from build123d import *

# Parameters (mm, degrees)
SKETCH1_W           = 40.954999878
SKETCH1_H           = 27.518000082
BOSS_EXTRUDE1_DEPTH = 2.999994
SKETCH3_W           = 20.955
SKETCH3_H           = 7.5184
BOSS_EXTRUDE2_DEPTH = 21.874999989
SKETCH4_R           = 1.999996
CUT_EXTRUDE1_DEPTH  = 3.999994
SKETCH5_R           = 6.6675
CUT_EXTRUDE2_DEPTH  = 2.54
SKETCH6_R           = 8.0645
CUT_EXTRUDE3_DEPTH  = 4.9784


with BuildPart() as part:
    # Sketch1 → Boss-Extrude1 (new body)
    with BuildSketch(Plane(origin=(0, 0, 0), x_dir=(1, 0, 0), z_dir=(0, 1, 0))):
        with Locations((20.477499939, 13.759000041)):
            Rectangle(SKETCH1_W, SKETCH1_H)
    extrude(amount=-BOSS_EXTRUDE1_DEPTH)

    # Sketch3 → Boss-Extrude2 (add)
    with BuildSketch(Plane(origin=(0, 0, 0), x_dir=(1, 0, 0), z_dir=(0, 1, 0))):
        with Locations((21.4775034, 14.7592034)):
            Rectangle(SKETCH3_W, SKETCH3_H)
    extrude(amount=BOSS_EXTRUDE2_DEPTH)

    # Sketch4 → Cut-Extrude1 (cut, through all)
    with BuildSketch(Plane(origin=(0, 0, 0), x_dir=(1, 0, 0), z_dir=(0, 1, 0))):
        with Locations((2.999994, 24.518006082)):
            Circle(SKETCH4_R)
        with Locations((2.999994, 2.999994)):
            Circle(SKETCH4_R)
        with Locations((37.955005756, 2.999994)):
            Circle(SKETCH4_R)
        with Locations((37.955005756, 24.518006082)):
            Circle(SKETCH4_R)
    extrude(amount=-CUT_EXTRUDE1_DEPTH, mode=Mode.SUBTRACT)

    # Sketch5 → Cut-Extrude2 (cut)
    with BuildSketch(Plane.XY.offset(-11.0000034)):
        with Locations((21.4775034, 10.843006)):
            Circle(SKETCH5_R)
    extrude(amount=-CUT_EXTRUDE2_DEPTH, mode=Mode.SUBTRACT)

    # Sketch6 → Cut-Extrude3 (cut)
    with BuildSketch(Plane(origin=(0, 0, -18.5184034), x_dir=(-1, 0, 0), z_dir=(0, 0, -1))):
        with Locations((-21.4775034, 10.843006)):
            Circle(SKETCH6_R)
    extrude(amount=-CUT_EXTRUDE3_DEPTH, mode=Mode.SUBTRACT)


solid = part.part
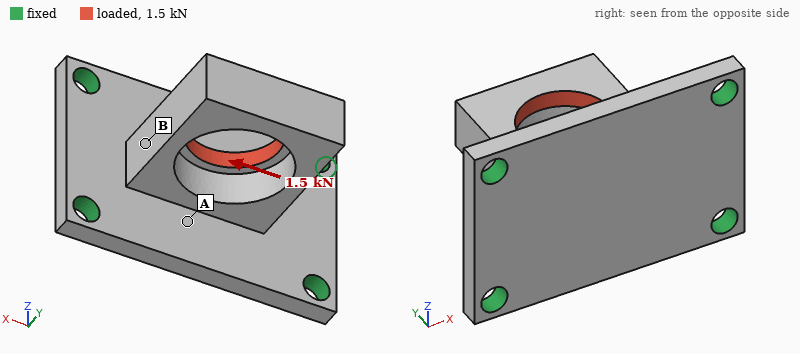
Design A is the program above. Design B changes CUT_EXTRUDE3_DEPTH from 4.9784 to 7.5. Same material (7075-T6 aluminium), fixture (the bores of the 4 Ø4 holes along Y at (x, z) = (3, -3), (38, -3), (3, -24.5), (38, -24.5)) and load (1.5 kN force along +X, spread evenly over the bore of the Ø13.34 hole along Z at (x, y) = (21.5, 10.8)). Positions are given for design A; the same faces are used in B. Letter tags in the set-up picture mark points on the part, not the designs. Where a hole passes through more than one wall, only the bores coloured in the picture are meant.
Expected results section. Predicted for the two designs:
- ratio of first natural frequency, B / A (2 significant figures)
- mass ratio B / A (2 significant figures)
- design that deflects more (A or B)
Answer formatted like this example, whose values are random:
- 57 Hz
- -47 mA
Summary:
- 1.0
- 0.97
- B
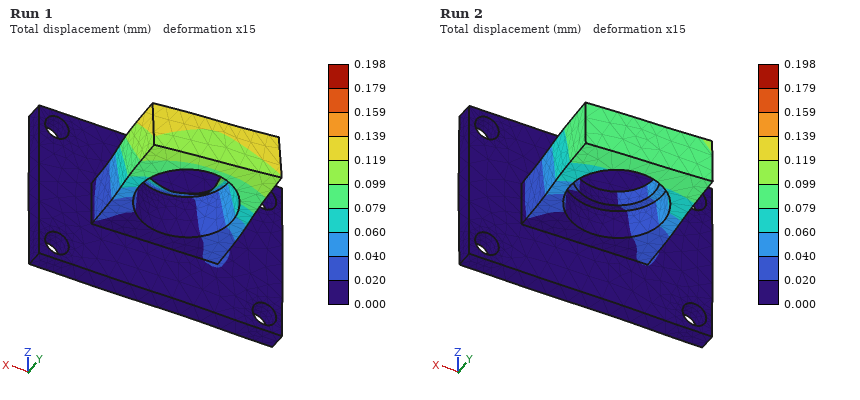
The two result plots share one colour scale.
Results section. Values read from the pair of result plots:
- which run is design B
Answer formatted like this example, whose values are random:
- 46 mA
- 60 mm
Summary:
- Run 1
